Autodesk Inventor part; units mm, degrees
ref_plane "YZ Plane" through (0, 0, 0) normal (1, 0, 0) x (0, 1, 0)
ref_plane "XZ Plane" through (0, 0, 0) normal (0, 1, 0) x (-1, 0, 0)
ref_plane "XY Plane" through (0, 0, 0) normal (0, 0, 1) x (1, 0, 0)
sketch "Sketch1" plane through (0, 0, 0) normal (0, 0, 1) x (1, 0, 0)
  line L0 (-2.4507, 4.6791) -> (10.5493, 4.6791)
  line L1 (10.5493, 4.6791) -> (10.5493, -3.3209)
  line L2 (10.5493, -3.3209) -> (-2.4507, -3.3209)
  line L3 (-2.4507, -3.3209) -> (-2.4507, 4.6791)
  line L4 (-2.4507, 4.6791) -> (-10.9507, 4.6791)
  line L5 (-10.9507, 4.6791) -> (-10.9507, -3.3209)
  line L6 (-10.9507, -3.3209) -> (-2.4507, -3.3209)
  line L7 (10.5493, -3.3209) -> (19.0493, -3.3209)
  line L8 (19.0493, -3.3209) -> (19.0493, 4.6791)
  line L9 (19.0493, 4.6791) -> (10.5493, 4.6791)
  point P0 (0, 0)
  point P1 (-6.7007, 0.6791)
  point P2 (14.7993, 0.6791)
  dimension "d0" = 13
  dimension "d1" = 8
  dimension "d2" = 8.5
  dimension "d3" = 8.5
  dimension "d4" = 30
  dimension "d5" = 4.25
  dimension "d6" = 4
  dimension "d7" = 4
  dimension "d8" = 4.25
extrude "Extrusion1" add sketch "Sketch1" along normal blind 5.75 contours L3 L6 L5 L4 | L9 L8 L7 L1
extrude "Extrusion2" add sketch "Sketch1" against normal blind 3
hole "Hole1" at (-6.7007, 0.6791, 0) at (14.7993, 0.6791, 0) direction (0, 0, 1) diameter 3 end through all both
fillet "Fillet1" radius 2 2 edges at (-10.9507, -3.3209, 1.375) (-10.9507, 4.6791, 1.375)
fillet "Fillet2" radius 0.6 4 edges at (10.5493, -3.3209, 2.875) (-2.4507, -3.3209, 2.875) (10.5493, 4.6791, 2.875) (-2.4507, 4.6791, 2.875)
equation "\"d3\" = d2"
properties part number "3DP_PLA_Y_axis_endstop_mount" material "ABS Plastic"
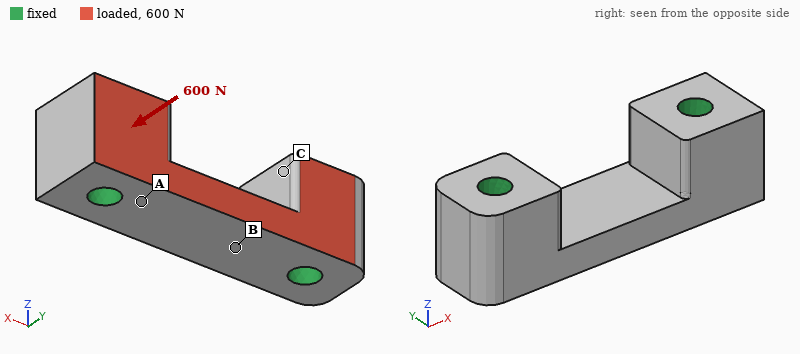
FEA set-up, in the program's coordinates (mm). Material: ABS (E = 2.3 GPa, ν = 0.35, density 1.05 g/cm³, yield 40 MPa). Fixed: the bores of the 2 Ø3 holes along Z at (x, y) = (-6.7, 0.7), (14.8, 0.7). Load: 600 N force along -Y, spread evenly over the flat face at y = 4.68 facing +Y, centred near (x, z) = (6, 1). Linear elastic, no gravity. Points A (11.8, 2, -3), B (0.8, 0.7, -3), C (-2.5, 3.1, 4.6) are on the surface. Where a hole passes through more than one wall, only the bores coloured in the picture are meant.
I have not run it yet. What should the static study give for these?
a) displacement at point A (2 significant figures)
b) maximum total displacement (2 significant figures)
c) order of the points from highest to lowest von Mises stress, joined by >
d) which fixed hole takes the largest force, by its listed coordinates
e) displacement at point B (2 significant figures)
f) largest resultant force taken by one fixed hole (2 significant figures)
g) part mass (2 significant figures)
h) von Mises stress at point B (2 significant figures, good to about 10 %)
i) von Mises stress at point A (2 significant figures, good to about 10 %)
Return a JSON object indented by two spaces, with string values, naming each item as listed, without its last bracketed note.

{
  "displacement at point A": "15 µm",
  "maximum total displacement": "53 µm",
  "order of the points from highest to lowest von Mises stress, joined by >": "A > B > C",
  "which fixed hole takes the largest force, by its listed coordinates": "(14.8, 0.7)",
  "displacement at point B": "43 µm",
  "largest resultant force taken by one fixed hole": "330 N",
  "part mass": "1.4 g",
  "von Mises stress at point B": "4.1 MPa",
  "von Mises stress at point A": "7.4 MPa"
}
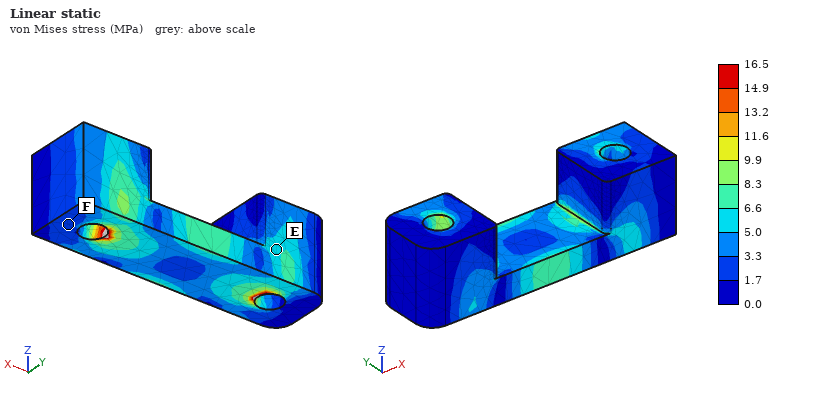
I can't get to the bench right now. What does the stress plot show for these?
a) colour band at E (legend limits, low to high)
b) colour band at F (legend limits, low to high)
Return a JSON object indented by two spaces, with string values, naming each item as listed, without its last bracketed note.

{
  "colour band at E": "5.0 to 6.6 MPa",
  "colour band at F": "1.7 to 3.3 MPa"
}
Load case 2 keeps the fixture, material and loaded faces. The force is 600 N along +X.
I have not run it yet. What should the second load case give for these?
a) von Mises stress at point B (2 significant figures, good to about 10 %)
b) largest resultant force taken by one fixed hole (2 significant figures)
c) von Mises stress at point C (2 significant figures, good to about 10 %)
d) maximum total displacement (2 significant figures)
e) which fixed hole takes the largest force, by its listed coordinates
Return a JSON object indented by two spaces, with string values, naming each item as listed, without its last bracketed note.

{
  "von Mises stress at point B": "3.9 MPa",
  "largest resultant force taken by one fixed hole": "330 N",
  "von Mises stress at point C": "4.2 MPa",
  "maximum total displacement": "40 µm",
  "which fixed hole takes the largest force, by its listed coordinates": "(14.8, 0.7)"
}
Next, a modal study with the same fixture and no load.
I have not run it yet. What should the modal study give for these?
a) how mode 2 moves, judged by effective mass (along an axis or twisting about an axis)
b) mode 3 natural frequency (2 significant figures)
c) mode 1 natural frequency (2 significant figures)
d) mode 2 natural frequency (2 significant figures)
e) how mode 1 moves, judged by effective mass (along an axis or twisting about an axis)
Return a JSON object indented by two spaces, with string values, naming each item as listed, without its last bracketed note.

{
  "how mode 2 moves, judged by effective mass": "along Y",
  "mode 3 natural frequency": "20 kHz",
  "mode 1 natural frequency": "15 kHz",
  "mode 2 natural frequency": "17 kHz",
  "how mode 1 moves, judged by effective mass": "along Z"
}
